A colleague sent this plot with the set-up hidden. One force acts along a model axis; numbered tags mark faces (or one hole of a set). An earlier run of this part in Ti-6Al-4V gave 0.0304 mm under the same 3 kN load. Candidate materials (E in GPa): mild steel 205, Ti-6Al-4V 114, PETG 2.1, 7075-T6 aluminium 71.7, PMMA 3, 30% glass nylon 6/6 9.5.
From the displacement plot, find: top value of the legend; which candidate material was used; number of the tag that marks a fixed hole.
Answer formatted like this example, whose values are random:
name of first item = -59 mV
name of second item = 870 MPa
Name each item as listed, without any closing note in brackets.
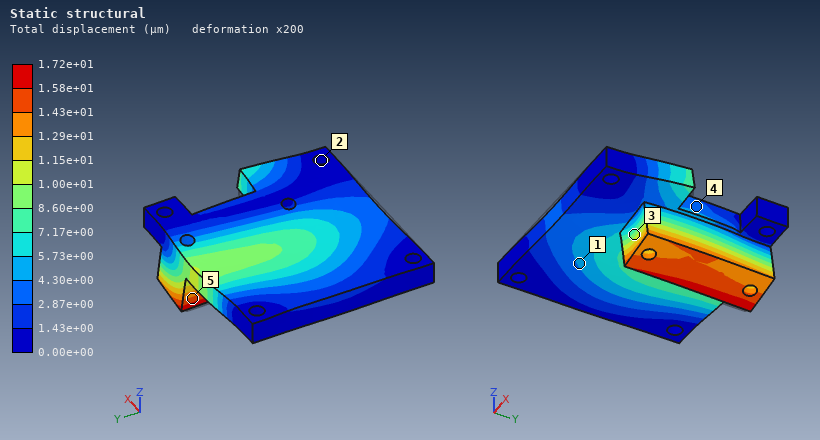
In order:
top value of the legend = 1.72e+01 µm
which candidate material was used = mild steel
number of the tag that marks a fixed hole = 2
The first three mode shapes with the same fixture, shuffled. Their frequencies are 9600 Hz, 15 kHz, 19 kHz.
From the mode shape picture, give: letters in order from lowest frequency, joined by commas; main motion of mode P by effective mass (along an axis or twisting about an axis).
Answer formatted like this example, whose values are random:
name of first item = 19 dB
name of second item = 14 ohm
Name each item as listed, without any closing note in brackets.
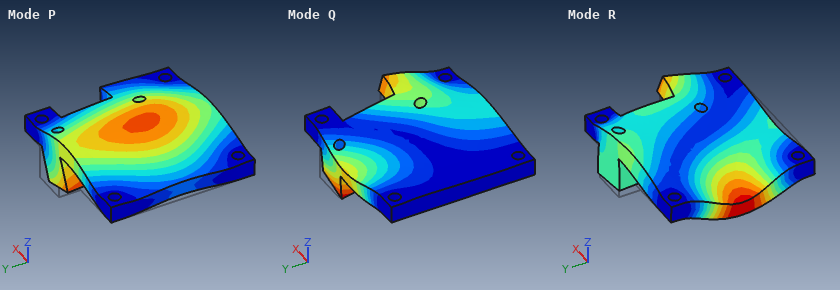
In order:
letters in order from lowest frequency, joined by commas = P, Q, R
main motion of mode P by effective mass = along Z
